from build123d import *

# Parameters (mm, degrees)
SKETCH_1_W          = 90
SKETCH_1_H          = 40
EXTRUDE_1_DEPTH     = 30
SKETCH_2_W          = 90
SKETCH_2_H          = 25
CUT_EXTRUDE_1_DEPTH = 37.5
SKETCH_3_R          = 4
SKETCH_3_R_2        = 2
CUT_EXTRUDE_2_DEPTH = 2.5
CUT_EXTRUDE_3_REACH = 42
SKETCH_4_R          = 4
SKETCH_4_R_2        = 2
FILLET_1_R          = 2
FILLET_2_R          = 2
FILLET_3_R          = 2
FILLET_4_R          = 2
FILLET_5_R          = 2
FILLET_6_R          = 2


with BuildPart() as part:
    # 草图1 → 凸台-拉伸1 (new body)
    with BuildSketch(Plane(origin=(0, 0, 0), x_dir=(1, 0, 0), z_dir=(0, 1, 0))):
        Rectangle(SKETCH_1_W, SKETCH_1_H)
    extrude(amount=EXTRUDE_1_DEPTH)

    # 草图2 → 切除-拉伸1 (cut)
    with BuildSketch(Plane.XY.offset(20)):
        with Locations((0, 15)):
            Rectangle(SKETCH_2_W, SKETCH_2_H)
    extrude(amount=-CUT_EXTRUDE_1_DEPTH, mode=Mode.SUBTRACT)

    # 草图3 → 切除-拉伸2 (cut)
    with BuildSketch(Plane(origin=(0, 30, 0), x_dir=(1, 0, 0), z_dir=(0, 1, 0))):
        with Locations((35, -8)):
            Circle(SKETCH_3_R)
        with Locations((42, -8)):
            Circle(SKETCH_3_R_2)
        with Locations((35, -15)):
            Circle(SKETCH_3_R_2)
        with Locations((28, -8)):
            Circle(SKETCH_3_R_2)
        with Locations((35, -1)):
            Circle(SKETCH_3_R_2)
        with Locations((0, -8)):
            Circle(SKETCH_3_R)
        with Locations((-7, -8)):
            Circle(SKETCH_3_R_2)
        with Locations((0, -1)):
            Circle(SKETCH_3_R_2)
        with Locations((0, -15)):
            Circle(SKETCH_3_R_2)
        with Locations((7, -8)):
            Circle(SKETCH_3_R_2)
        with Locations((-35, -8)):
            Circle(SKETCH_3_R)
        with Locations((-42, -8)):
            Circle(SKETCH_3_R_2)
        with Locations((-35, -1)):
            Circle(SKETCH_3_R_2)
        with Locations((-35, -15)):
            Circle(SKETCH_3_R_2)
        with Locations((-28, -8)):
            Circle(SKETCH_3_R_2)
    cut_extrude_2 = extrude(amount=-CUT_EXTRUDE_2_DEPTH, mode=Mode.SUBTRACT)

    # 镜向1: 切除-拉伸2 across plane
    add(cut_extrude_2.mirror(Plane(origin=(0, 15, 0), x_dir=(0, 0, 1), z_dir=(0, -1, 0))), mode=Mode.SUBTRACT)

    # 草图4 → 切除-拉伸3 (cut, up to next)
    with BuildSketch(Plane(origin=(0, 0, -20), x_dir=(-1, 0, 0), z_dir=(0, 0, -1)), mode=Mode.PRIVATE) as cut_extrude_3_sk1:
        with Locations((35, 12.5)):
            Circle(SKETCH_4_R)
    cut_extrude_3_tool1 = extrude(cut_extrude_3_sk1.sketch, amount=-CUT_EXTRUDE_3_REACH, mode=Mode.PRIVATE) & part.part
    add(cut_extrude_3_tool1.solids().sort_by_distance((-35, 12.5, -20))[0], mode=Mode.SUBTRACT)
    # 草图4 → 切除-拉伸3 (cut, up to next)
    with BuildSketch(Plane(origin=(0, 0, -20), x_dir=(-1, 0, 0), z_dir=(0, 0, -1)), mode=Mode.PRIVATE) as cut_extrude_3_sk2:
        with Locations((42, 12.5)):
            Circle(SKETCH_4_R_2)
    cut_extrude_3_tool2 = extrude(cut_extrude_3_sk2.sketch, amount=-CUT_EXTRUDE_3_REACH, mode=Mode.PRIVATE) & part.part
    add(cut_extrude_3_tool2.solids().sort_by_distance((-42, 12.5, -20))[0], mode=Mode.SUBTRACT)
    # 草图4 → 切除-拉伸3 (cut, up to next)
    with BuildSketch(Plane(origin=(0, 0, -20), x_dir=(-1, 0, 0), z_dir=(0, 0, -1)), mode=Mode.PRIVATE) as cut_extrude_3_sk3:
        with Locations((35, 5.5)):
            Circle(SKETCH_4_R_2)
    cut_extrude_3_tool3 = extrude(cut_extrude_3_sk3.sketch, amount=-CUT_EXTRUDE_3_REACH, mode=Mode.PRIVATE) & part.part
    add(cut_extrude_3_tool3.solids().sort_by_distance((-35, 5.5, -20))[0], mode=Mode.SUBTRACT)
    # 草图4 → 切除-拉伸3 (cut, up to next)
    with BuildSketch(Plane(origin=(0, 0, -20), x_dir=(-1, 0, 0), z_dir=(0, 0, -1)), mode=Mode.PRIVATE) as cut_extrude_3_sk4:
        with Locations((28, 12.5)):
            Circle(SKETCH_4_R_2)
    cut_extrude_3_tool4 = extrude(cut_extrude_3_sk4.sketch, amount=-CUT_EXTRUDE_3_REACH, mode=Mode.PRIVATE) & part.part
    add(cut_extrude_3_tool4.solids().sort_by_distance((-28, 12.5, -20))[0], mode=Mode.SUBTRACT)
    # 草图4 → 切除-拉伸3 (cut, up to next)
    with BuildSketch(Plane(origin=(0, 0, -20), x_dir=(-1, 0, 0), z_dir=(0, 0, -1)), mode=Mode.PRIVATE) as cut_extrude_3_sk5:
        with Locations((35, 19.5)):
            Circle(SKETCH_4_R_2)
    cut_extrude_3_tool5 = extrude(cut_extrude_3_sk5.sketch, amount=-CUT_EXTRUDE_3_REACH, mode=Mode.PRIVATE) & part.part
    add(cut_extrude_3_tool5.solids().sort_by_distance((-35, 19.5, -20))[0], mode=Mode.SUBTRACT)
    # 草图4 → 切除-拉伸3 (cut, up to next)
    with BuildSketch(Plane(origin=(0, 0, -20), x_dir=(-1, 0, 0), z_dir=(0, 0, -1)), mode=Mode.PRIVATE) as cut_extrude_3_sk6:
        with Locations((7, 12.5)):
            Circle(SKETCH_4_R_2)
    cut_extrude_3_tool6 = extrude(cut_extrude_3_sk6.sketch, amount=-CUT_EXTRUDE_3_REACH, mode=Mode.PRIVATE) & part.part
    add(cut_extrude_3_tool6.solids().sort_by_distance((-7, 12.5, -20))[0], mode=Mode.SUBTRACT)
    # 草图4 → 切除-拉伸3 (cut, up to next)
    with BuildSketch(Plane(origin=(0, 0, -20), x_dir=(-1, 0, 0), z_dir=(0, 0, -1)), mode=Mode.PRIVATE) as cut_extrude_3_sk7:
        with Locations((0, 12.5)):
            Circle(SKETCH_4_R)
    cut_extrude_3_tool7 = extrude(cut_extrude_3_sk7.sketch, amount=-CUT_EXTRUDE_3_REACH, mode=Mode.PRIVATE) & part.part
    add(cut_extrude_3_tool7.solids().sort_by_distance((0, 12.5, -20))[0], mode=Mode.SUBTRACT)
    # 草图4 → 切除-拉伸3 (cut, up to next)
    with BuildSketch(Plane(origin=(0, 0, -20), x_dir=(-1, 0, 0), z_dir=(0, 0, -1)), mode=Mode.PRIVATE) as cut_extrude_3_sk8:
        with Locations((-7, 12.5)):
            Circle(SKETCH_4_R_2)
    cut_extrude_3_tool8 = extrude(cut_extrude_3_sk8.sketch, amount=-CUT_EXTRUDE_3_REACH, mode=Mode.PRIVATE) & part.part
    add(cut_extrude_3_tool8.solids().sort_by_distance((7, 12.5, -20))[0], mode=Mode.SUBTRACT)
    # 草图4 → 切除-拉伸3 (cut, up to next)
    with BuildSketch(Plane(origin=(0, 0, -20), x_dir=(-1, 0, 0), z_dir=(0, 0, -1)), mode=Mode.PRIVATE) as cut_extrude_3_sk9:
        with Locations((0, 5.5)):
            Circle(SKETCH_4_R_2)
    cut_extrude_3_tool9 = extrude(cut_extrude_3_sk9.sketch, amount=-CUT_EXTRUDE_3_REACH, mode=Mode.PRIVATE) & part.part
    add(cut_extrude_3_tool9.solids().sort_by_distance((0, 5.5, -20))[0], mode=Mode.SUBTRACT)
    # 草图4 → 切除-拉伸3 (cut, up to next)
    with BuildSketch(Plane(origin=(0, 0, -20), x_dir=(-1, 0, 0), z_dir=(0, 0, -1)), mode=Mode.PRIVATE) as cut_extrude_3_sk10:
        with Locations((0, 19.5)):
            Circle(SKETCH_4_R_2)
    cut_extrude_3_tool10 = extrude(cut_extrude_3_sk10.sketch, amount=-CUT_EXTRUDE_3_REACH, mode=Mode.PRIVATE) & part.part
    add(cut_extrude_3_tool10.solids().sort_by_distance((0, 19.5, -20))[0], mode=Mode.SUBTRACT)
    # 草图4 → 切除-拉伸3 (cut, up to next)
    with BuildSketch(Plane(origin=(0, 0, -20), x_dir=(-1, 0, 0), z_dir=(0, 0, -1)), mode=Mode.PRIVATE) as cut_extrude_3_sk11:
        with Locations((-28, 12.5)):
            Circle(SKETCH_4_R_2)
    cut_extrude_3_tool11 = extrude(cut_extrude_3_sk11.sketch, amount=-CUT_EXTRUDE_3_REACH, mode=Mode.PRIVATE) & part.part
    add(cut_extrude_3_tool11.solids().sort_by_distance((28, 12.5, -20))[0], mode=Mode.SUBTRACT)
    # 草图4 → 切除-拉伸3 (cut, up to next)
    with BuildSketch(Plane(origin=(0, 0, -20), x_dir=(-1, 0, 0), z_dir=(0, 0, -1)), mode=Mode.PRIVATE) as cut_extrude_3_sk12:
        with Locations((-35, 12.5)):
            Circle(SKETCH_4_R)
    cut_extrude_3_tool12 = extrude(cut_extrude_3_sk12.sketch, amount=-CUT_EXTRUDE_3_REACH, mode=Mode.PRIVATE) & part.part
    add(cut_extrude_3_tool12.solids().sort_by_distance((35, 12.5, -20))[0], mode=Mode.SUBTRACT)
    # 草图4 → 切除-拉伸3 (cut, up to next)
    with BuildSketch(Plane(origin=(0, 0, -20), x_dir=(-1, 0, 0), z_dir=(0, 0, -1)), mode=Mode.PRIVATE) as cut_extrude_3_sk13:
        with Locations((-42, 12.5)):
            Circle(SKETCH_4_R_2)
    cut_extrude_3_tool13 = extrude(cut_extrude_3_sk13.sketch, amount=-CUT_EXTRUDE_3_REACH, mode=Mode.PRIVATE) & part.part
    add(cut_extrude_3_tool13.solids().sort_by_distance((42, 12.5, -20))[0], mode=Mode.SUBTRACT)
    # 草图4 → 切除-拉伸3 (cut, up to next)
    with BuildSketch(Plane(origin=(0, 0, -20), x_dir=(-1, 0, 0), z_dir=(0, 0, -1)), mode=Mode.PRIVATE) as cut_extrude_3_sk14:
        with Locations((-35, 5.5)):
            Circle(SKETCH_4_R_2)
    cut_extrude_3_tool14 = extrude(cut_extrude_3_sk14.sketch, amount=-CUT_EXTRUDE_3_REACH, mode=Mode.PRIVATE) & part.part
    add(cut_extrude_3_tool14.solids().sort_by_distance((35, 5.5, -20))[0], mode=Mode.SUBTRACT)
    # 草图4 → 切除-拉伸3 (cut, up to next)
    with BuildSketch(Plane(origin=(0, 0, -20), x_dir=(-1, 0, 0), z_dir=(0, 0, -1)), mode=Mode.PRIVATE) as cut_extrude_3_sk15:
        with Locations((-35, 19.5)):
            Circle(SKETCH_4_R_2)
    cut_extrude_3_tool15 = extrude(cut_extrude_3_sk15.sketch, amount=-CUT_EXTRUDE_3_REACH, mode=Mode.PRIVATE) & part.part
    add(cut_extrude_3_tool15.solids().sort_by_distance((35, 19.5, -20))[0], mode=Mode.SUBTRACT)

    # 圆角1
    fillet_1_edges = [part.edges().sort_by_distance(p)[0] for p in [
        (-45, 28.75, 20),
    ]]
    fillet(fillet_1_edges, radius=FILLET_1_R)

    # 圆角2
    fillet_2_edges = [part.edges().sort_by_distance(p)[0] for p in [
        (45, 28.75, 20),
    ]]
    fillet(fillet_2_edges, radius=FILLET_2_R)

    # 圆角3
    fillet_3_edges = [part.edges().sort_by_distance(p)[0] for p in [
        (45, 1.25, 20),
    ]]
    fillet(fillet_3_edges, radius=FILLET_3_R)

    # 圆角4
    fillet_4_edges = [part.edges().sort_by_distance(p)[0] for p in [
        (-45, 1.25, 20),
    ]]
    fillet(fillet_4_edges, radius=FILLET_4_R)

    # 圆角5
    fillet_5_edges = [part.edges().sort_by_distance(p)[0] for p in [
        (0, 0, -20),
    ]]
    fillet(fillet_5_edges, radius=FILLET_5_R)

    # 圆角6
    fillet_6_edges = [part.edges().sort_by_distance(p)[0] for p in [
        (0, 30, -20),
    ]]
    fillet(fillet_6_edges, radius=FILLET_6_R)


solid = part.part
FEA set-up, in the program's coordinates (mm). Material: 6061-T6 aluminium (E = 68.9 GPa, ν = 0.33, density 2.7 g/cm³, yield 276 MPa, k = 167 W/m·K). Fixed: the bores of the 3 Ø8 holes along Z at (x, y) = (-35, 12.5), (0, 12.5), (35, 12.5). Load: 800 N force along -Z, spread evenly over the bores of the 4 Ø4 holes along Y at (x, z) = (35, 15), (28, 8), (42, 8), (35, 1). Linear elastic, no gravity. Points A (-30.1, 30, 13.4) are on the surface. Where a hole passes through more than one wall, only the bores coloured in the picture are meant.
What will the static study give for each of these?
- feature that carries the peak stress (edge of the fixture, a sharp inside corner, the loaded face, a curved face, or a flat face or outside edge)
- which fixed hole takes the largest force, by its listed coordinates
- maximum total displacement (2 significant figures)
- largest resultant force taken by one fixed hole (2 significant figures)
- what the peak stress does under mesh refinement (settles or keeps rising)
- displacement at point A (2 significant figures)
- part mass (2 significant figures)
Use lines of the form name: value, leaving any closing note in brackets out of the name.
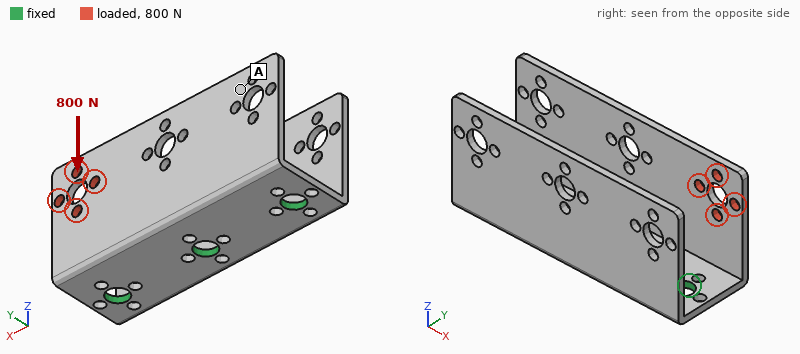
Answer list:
feature that carries the peak stress: a sharp inside corner
which fixed hole takes the largest force, by its listed coordinates: (35, 12.5)
maximum total displacement: 0.86 mm
largest resultant force taken by one fixed hole: 640 N
what the peak stress does under mesh refinement: keeps rising
displacement at point A: 0.22 mm
part mass: 57 g
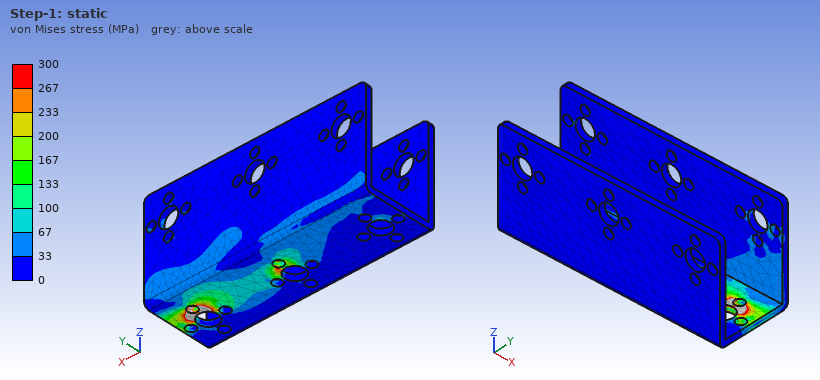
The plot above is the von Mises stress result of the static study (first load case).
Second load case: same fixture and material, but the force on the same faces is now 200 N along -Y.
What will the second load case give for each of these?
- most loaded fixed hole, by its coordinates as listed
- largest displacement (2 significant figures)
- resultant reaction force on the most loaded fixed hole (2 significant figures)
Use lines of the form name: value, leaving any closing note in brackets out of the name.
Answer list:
most loaded fixed hole, by its coordinates as listed: (35, 12.5)
largest displacement: 1.2 mm
resultant reaction force on the most loaded fixed hole: 180 N
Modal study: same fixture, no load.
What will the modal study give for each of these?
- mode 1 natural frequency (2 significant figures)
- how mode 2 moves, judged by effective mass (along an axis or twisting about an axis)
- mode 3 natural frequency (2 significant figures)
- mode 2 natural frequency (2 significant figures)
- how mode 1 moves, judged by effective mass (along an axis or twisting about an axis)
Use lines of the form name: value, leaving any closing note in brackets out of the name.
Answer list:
mode 1 natural frequency: 900 Hz
how mode 2 moves, judged by effective mass: along Y
mode 3 natural frequency: 1500 Hz
mode 2 natural frequency: 1000 Hz
how mode 1 moves, judged by effective mass: along Y
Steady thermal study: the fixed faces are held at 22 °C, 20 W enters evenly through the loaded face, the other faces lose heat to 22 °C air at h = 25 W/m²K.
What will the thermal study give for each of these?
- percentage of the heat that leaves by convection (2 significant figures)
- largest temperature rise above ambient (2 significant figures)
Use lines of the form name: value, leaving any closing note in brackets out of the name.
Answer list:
percentage of the heat that leaves by convection: 18 %
largest temperature rise above ambient: 54 K
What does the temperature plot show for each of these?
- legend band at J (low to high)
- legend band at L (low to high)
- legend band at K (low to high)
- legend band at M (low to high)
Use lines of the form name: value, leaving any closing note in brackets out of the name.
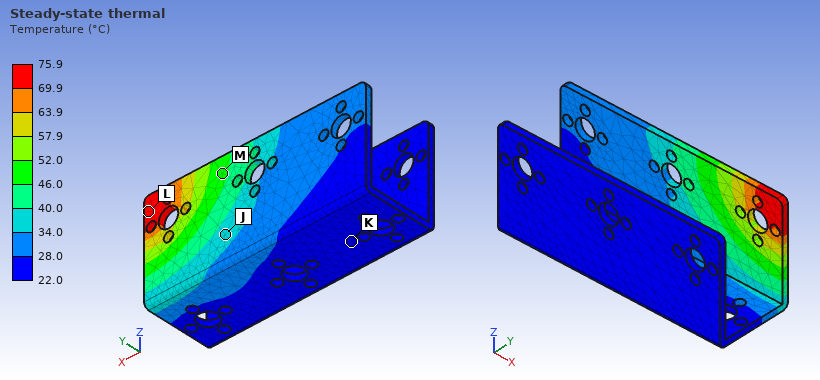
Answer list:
legend band at J: 34.0 to 40.0 °C
legend band at L: 69.9 to 75.9 °C
legend band at K: 22.0 to 28.0 °C
legend band at M: 46.0 to 52.0 °C
